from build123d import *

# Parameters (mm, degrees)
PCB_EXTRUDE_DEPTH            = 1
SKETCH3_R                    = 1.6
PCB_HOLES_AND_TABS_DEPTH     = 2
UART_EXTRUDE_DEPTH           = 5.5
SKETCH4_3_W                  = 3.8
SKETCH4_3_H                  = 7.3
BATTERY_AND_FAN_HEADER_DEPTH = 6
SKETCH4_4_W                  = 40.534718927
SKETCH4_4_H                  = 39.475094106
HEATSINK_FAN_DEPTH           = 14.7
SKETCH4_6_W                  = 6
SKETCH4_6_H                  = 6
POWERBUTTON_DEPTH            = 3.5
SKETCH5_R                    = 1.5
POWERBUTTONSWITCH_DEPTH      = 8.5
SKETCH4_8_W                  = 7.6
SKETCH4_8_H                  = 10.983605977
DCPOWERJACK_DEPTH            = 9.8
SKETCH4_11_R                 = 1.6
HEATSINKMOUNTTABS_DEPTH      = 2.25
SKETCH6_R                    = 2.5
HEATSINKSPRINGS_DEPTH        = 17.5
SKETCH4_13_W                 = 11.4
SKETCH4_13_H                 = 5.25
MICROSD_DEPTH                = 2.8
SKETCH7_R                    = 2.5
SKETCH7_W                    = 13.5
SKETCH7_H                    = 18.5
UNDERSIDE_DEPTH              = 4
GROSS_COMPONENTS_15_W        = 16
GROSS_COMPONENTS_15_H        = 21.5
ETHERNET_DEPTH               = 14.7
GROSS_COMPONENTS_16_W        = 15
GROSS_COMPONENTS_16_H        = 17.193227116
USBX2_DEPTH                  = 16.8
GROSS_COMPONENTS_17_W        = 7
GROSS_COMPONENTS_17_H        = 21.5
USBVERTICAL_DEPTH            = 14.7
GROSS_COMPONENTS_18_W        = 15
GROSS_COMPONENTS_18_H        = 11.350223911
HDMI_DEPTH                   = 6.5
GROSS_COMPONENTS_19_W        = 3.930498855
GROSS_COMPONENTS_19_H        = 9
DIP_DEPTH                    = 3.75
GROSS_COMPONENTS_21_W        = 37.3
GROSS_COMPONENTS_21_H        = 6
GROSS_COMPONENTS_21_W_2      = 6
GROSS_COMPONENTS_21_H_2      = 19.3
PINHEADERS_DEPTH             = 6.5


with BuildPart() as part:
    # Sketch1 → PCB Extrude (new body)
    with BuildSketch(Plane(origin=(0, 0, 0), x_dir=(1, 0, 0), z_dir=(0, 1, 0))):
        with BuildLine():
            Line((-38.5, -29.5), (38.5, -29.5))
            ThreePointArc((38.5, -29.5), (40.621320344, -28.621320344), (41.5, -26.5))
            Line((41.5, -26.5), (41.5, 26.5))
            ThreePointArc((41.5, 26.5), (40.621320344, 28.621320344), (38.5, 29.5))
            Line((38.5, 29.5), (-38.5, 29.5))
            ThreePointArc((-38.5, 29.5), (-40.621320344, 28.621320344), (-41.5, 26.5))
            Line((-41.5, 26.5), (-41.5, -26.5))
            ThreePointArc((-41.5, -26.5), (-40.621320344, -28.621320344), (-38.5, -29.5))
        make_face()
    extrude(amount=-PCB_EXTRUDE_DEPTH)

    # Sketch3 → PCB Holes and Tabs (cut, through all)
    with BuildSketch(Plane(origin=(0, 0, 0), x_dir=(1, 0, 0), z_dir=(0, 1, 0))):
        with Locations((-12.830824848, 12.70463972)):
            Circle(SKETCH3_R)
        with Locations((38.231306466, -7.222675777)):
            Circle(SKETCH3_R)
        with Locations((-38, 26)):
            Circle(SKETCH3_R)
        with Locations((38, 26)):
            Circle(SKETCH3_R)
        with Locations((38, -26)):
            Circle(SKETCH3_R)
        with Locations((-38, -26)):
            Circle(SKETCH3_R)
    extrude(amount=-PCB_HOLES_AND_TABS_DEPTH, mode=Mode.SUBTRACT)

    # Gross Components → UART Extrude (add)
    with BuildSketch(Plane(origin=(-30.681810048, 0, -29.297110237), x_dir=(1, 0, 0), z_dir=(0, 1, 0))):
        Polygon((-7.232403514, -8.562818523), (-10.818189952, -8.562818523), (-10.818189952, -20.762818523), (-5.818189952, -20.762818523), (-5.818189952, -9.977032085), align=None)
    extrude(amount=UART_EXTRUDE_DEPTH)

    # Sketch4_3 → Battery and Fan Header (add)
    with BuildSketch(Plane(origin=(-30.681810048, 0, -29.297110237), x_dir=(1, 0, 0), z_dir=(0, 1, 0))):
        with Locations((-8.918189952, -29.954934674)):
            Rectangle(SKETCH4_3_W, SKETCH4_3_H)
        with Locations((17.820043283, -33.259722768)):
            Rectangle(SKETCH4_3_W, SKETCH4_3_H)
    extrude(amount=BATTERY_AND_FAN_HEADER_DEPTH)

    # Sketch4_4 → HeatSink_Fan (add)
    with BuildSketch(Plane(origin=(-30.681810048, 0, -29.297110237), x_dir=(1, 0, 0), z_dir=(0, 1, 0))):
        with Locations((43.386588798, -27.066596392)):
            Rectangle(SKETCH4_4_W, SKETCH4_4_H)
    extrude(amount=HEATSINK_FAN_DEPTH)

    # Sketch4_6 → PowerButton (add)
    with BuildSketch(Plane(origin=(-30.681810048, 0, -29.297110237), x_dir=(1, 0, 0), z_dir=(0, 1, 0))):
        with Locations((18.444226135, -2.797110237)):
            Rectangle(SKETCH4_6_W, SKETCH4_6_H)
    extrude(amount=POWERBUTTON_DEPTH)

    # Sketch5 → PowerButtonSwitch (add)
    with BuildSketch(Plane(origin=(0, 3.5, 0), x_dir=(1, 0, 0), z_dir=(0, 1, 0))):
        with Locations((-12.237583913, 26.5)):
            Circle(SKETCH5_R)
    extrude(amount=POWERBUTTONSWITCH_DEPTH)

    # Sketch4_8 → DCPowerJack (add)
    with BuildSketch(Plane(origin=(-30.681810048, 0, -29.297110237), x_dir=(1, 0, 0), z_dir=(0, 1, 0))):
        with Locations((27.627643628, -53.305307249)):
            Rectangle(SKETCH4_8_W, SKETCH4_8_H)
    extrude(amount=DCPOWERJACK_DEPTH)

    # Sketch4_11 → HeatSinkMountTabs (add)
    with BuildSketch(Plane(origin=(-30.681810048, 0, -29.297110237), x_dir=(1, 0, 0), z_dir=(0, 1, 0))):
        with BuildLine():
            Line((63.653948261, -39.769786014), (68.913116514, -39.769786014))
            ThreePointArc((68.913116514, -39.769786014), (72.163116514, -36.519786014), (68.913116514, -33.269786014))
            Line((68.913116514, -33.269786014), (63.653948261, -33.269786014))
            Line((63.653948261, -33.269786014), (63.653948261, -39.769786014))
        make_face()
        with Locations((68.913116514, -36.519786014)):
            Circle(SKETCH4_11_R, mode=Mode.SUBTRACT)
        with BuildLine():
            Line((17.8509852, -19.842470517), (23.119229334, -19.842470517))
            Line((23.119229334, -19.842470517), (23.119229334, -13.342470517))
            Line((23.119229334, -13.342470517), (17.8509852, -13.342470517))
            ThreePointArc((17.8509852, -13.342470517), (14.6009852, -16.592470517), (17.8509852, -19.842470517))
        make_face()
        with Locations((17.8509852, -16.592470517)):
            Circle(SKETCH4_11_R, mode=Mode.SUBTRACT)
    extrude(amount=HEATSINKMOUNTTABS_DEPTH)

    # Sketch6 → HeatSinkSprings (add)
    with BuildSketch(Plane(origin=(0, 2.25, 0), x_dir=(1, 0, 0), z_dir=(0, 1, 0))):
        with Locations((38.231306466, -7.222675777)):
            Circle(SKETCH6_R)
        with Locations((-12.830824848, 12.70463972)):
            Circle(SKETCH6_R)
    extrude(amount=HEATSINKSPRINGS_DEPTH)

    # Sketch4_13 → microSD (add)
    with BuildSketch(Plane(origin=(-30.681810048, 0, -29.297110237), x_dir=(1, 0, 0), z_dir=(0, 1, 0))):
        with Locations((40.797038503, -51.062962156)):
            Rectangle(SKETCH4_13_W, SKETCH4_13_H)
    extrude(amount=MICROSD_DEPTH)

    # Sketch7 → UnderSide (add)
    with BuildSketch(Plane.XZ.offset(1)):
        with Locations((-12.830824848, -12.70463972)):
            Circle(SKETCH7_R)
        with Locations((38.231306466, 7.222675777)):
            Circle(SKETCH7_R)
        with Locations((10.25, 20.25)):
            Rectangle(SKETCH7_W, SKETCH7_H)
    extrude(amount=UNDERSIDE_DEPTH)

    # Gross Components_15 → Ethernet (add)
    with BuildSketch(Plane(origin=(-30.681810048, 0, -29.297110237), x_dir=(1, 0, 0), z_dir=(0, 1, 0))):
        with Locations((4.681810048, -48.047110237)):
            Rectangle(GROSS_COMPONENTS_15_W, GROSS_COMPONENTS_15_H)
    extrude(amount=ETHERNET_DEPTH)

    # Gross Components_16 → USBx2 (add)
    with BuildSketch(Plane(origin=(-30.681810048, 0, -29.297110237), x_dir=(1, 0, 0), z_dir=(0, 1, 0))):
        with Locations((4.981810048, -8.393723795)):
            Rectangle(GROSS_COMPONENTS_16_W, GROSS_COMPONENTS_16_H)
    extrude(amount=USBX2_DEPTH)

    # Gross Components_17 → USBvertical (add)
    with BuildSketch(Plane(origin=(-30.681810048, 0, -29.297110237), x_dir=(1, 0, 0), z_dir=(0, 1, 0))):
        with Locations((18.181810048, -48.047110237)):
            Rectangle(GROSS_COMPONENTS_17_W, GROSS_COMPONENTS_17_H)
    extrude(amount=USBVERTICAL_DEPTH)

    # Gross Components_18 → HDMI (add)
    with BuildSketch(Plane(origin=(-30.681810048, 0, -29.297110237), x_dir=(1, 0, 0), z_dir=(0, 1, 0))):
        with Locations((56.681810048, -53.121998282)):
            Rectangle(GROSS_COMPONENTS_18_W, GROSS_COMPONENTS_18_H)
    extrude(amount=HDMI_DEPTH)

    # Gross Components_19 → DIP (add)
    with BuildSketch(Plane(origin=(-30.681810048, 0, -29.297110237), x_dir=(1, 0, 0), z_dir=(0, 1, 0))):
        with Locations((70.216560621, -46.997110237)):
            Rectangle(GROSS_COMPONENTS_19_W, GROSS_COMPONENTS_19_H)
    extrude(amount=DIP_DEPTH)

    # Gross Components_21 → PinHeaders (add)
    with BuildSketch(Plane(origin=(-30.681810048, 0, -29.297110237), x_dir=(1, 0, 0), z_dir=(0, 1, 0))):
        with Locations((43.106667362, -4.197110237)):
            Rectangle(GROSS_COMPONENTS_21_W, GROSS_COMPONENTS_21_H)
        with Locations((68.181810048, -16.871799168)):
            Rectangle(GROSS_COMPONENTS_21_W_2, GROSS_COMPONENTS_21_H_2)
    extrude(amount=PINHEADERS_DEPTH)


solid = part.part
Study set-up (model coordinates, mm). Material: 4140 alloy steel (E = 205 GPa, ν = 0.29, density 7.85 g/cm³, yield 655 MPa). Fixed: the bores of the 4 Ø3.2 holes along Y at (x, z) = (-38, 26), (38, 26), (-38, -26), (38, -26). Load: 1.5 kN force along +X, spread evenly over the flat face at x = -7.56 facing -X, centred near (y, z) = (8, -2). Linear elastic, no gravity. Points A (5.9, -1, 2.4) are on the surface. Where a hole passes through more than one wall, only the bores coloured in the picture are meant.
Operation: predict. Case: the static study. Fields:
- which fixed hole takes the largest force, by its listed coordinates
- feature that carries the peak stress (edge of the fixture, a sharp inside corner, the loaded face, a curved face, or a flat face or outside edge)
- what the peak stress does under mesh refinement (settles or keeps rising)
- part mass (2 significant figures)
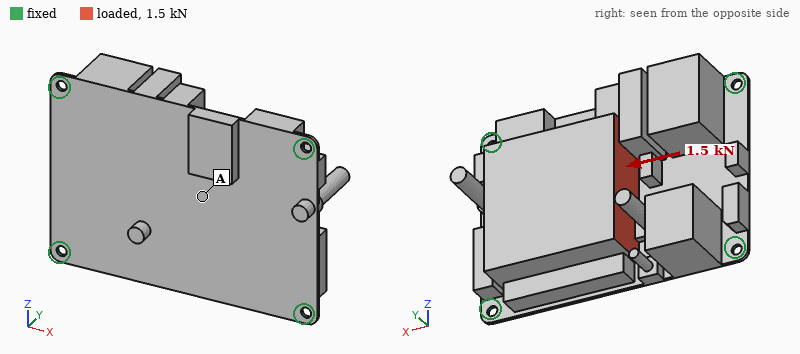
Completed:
(-38, 26)
edge of the fixture
keeps rising
370 g
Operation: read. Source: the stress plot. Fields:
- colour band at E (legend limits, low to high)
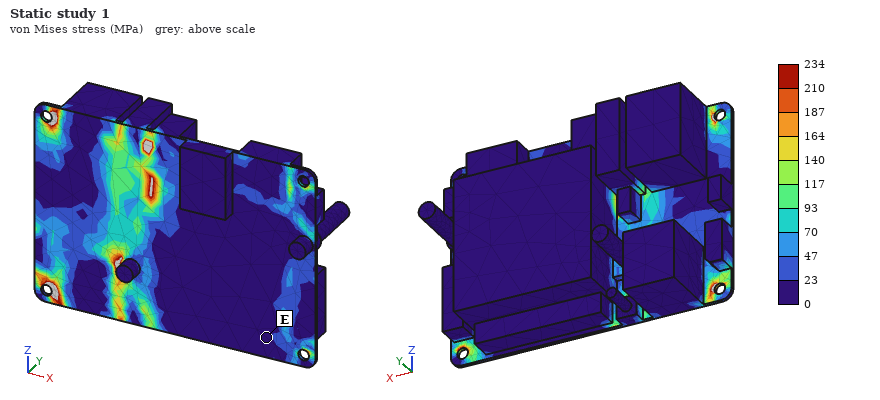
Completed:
0 to 23 MPa
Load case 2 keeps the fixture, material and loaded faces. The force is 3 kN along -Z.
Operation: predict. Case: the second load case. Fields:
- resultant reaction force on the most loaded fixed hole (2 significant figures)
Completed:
1.3 kN
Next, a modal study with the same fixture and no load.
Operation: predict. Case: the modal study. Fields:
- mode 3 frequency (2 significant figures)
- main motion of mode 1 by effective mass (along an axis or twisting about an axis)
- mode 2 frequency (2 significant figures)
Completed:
2000 Hz
along Y
1800 Hz
